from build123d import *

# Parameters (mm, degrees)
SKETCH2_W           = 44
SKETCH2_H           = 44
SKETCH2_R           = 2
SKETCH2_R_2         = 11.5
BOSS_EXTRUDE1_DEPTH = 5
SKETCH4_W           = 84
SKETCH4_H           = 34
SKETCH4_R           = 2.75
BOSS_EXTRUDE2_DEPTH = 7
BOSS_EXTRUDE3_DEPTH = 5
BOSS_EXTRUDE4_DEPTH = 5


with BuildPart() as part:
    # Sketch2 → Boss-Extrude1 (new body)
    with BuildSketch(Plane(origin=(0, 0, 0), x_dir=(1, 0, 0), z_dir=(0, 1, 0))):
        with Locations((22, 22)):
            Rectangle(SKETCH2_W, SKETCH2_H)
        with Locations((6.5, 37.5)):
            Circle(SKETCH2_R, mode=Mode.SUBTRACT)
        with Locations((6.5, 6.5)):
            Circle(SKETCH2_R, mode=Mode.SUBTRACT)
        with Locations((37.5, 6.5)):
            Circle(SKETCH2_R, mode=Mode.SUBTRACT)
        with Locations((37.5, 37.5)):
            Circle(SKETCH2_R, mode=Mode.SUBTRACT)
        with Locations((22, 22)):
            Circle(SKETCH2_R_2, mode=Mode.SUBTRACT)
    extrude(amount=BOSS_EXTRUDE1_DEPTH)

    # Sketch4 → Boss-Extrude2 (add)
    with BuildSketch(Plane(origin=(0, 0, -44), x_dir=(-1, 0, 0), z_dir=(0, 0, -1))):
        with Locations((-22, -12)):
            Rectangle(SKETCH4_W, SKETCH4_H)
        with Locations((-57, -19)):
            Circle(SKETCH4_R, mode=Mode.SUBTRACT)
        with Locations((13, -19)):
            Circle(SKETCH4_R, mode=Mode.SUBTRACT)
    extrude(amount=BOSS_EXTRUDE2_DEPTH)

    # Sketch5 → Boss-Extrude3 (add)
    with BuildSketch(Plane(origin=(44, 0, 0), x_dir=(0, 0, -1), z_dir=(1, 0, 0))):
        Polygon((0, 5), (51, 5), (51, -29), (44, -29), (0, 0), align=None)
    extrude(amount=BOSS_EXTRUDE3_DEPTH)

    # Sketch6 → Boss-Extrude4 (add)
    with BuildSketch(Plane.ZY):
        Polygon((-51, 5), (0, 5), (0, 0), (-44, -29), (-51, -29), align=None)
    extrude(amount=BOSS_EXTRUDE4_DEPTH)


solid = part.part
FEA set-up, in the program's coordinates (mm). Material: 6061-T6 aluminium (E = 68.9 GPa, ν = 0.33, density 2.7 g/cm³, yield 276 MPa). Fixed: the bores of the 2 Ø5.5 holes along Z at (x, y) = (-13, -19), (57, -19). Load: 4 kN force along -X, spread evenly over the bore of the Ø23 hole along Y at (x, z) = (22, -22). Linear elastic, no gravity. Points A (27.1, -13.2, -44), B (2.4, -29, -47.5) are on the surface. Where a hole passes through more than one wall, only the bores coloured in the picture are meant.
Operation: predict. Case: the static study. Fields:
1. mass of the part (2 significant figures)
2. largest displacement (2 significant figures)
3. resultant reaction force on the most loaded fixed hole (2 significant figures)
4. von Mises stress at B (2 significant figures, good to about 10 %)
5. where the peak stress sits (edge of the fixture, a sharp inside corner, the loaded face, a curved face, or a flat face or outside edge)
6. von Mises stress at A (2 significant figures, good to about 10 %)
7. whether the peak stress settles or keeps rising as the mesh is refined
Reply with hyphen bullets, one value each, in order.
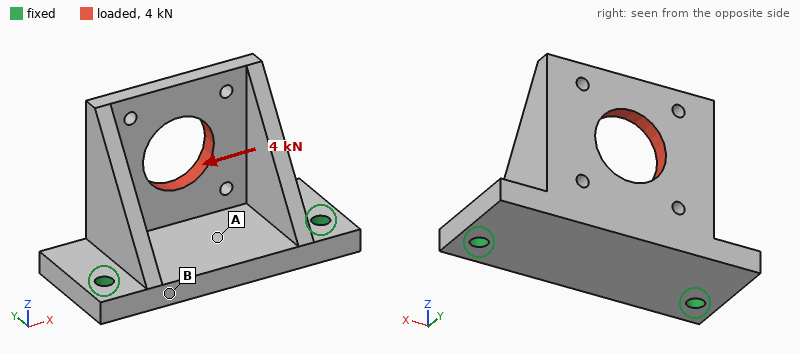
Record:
- 96 g
- 0.17 mm
- 2.8 kN
- 14 MPa
- edge of the fixture
- 33 MPa
- keeps rising
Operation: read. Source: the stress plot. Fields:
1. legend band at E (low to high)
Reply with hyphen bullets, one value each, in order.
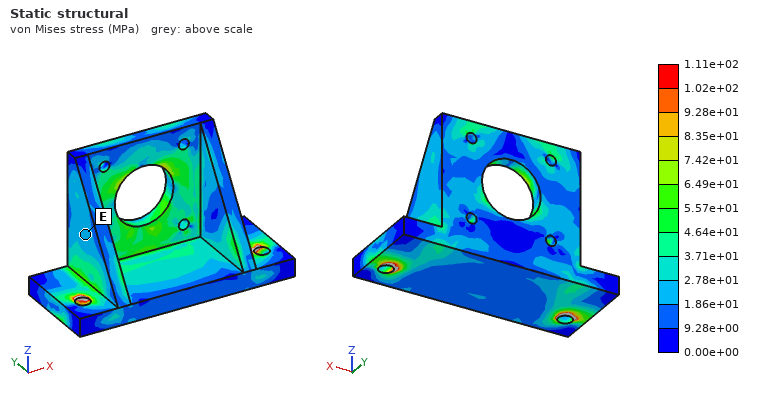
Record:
- 1.86e+01 to 2.78e+01 MPa
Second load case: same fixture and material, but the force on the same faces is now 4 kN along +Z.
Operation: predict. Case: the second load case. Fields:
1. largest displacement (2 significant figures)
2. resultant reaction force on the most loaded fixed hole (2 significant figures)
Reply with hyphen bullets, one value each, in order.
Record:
- 0.35 mm
- 2.0 kN
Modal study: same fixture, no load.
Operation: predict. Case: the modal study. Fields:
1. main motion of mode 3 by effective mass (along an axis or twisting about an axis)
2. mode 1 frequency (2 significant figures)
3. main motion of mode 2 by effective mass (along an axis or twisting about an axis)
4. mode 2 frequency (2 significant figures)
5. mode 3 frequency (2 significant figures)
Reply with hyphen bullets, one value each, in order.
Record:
- along Z
- 2500 Hz
- along X
- 4100 Hz
- 7200 Hz
